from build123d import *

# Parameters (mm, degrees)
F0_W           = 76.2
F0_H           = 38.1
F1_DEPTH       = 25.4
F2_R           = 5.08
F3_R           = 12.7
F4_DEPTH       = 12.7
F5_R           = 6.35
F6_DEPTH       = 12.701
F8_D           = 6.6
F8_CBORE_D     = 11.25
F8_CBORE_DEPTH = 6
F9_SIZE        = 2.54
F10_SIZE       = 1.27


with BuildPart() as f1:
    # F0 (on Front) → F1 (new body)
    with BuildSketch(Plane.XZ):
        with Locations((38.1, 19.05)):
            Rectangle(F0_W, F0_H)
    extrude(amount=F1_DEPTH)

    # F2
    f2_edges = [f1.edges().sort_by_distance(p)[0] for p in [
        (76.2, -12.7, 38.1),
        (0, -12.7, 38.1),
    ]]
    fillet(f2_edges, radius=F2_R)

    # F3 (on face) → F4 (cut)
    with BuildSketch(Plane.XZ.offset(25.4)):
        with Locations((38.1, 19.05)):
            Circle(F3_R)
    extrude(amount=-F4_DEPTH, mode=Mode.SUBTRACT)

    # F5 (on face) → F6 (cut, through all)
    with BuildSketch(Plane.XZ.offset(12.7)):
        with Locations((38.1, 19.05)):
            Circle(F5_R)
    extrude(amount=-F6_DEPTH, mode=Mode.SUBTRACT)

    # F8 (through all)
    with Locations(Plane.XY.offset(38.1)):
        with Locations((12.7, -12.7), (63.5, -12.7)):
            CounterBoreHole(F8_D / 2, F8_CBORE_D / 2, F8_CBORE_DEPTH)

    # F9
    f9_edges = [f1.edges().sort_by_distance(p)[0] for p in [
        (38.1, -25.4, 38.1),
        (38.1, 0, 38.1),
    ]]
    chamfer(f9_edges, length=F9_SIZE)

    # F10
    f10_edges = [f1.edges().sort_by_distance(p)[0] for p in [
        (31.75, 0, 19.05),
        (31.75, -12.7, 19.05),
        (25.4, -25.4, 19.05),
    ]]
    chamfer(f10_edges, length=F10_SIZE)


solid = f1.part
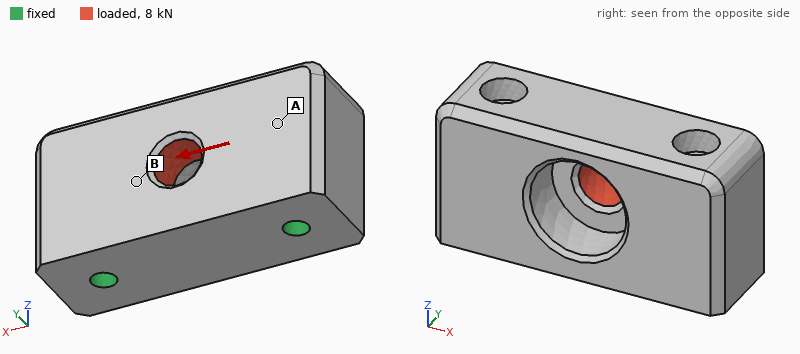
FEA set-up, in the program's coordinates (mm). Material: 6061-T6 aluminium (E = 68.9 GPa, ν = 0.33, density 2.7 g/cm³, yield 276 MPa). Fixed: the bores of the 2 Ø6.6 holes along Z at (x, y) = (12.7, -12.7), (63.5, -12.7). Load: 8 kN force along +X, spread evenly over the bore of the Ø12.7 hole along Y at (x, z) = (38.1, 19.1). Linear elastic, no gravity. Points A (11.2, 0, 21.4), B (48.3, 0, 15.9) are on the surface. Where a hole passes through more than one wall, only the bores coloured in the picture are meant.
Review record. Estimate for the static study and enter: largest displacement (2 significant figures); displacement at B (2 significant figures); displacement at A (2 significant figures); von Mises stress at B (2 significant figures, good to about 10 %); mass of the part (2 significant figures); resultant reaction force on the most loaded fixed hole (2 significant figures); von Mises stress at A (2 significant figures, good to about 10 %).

4.5 µm
3.1 µm
1.3 µm
12 MPa
160 g
4.1 kN
3.5 MPa
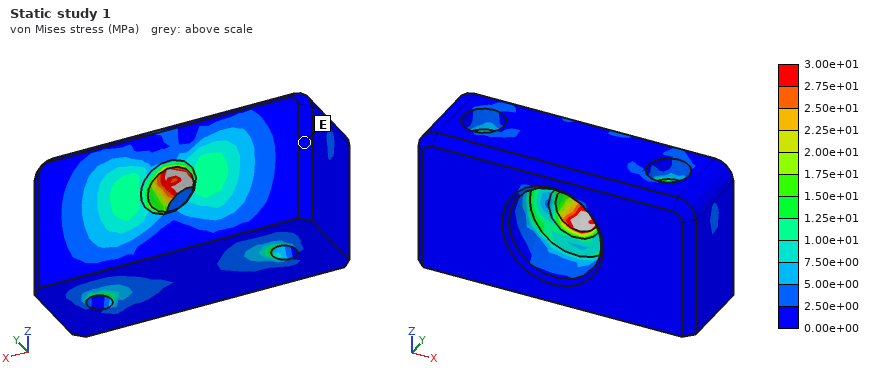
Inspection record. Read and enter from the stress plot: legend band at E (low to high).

0.00e+00 to 2.50e+00 MPa
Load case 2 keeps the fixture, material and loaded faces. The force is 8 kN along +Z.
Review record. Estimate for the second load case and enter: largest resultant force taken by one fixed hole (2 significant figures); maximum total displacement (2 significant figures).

4.0 kN
9.4 µm
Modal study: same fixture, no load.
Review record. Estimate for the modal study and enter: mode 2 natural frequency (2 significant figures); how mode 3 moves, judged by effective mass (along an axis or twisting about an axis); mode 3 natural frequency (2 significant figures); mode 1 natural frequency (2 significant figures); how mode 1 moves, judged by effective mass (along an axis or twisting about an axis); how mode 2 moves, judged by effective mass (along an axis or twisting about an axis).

25 kHz
along Z
28 kHz
19 kHz
along Y
twisting about X
